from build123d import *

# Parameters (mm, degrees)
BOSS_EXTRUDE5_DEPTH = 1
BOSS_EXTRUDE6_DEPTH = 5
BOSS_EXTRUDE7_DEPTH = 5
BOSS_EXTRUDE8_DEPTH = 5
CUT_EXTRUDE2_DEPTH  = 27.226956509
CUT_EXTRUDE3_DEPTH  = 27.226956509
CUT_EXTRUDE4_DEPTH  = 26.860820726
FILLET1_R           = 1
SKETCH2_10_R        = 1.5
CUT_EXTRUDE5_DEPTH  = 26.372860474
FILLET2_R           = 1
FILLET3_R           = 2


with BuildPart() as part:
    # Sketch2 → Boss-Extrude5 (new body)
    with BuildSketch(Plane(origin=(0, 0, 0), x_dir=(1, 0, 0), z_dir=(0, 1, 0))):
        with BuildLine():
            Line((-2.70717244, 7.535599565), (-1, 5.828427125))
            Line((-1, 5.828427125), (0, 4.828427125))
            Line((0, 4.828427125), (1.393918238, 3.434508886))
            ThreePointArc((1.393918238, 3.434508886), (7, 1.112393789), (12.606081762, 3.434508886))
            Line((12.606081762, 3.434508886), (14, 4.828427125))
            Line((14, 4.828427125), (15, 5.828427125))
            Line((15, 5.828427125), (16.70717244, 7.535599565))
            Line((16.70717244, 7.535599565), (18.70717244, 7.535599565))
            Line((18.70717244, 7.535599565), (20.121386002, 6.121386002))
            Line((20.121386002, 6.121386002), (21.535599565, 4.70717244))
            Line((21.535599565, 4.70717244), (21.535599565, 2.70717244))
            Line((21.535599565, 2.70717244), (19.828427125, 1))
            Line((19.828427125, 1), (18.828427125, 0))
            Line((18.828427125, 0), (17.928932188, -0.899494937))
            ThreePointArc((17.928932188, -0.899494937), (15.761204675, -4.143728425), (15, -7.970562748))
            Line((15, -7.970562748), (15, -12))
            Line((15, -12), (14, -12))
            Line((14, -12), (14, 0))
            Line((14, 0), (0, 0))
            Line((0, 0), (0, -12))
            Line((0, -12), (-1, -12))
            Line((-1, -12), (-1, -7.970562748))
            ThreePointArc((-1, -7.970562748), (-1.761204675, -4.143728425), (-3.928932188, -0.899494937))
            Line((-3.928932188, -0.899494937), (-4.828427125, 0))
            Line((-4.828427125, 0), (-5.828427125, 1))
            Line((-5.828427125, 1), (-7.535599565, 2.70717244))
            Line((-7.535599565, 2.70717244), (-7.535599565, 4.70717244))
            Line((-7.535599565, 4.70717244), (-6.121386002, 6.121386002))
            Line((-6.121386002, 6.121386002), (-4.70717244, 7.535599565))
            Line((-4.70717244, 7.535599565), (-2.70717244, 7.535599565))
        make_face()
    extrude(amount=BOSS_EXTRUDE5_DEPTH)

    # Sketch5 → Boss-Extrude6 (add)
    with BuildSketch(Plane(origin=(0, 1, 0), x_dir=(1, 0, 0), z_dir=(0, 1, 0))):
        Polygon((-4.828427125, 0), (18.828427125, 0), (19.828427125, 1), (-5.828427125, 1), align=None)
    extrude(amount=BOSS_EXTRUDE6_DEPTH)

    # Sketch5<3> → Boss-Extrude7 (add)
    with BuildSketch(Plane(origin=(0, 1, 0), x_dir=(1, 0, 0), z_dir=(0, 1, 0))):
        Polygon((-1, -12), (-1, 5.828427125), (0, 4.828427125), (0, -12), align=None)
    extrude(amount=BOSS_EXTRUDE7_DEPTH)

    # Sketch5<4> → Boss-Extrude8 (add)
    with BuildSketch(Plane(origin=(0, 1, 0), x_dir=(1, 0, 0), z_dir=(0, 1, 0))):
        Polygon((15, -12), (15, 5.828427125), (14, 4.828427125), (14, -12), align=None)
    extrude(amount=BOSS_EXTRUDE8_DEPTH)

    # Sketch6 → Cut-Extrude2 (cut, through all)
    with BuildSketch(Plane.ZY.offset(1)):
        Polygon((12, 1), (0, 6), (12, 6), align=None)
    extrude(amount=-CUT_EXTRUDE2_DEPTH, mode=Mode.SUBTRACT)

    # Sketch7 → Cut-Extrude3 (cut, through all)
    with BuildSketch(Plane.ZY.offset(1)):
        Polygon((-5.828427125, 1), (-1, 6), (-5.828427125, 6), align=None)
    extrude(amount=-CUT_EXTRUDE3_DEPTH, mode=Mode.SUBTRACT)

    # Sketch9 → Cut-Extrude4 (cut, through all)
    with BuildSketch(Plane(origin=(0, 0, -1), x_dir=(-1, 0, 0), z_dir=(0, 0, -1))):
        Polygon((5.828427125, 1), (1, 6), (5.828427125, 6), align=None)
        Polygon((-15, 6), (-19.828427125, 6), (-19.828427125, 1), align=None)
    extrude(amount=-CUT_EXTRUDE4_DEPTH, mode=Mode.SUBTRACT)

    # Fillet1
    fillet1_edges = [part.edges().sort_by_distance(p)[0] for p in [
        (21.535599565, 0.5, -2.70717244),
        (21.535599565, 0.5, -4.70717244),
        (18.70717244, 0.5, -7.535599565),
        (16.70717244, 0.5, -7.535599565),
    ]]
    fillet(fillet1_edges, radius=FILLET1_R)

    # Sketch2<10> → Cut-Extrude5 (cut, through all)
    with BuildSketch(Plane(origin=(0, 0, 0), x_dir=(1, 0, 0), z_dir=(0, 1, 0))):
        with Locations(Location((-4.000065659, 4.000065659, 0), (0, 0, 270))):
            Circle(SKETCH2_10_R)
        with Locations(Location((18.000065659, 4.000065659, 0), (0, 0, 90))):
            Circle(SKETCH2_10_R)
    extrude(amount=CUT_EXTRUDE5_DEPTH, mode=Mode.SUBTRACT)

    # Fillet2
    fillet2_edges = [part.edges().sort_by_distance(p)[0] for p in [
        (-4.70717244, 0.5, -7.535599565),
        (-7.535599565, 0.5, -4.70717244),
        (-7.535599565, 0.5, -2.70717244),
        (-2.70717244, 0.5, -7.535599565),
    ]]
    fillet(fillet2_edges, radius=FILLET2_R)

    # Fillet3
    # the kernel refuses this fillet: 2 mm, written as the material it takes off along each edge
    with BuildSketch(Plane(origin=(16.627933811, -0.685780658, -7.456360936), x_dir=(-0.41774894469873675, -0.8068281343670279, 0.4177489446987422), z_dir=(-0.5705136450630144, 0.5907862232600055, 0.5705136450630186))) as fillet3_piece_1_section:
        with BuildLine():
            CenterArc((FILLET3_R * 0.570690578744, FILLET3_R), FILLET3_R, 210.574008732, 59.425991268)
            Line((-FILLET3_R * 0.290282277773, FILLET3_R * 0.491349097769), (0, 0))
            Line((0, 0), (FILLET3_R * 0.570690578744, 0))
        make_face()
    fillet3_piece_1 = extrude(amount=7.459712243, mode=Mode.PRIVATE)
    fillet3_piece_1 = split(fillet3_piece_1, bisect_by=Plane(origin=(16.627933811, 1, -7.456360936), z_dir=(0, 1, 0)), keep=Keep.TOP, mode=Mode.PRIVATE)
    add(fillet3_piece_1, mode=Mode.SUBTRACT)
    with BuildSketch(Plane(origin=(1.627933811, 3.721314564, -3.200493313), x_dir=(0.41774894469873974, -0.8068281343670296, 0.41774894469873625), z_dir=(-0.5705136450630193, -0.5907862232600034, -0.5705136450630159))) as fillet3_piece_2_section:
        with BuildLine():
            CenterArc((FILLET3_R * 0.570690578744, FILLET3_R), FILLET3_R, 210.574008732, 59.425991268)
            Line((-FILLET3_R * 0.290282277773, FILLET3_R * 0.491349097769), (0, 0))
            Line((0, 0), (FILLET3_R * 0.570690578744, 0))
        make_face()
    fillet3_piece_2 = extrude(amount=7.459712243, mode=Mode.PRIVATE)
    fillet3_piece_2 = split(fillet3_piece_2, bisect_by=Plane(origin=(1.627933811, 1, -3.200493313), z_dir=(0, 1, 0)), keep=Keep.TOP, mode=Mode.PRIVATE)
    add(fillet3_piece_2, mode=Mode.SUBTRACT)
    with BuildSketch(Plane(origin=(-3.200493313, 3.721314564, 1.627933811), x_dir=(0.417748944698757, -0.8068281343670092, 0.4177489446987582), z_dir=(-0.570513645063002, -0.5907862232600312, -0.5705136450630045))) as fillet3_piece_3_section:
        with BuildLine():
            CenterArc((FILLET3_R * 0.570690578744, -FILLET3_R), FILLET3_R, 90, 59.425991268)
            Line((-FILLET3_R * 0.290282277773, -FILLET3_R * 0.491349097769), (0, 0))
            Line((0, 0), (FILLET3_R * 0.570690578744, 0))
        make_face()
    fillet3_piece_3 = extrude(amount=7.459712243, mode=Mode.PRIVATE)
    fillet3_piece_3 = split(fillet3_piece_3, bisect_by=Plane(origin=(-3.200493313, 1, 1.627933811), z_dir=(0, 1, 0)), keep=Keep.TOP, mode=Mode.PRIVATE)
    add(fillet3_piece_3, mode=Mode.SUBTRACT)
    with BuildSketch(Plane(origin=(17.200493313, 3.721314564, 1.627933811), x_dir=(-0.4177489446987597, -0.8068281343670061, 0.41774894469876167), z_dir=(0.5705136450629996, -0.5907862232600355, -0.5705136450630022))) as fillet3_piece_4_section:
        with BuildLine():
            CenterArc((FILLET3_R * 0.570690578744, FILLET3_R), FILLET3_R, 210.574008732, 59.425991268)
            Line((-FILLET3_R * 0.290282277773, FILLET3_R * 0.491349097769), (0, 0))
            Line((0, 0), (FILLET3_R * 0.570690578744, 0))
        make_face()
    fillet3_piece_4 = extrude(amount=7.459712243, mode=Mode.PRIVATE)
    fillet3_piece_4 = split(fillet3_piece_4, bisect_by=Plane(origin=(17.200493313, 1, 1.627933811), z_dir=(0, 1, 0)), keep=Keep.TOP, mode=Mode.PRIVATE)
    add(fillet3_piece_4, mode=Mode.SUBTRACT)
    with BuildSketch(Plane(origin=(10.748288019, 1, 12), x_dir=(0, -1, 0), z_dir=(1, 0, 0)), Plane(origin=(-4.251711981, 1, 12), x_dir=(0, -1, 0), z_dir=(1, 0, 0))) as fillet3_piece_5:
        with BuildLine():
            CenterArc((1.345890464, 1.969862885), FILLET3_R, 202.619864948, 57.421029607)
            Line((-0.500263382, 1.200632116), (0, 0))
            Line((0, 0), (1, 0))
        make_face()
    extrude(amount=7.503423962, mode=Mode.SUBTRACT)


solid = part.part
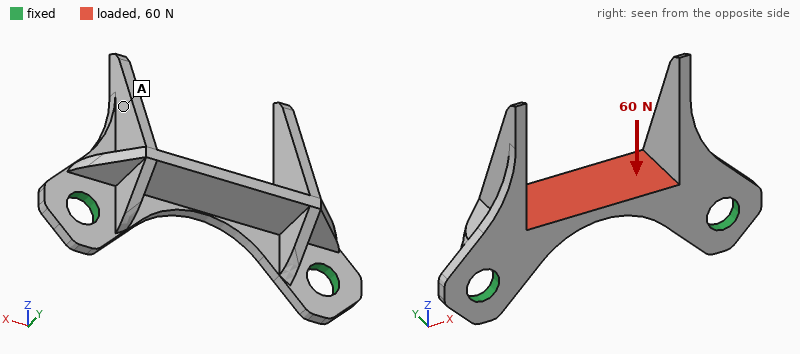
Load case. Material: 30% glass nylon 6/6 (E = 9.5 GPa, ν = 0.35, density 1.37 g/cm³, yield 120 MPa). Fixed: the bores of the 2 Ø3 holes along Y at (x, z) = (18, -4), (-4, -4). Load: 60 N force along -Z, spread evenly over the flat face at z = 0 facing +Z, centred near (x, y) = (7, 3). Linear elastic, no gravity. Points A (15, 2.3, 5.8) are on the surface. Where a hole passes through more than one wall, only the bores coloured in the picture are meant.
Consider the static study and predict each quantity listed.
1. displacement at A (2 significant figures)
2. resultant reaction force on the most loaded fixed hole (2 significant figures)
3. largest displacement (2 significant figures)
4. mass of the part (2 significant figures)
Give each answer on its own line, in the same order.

0.10 mm
34 N
0.18 mm
0.46 g
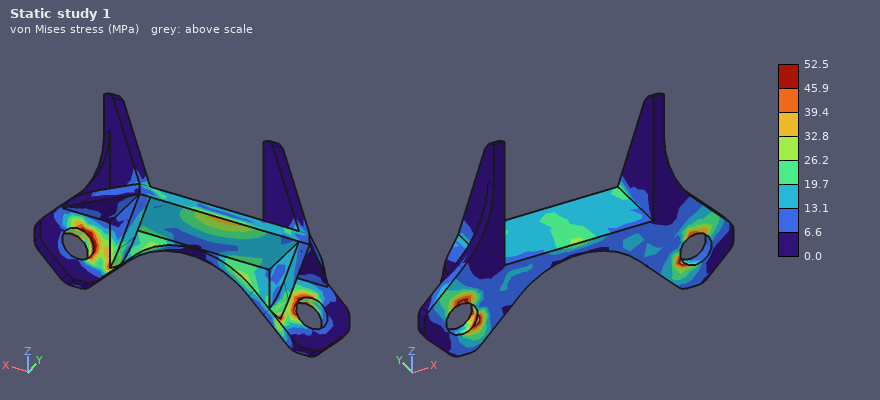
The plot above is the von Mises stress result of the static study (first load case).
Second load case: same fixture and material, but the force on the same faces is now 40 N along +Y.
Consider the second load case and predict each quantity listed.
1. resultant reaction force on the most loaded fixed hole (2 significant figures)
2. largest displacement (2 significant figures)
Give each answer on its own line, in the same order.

28 N
0.13 mm
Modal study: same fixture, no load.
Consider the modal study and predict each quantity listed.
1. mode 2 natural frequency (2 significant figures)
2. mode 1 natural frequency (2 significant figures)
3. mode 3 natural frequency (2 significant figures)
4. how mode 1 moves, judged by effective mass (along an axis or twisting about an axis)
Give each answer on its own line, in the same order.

6900 Hz
5300 Hz
7800 Hz
along Y
